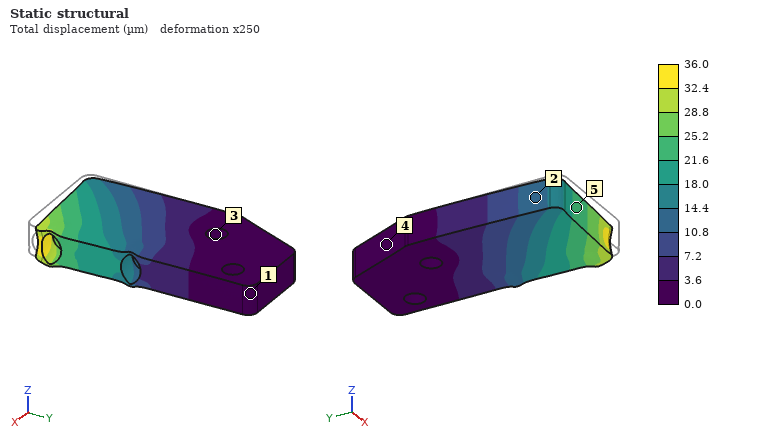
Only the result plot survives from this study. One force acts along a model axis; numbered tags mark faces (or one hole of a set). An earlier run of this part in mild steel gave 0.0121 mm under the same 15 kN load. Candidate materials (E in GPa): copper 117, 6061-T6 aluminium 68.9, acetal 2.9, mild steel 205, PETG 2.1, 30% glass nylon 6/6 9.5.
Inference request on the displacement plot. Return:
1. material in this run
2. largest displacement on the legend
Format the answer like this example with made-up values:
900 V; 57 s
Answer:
6061-T6 aluminium; 36.0 µm
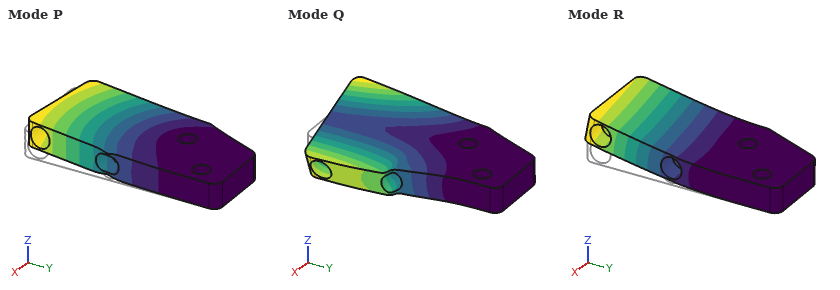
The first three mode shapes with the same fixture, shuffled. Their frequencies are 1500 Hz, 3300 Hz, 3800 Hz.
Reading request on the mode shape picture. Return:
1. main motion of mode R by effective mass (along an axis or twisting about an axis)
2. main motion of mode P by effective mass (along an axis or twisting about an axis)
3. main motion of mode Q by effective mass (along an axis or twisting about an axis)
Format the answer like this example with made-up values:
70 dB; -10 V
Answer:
along Z; along X; twisting about Y
